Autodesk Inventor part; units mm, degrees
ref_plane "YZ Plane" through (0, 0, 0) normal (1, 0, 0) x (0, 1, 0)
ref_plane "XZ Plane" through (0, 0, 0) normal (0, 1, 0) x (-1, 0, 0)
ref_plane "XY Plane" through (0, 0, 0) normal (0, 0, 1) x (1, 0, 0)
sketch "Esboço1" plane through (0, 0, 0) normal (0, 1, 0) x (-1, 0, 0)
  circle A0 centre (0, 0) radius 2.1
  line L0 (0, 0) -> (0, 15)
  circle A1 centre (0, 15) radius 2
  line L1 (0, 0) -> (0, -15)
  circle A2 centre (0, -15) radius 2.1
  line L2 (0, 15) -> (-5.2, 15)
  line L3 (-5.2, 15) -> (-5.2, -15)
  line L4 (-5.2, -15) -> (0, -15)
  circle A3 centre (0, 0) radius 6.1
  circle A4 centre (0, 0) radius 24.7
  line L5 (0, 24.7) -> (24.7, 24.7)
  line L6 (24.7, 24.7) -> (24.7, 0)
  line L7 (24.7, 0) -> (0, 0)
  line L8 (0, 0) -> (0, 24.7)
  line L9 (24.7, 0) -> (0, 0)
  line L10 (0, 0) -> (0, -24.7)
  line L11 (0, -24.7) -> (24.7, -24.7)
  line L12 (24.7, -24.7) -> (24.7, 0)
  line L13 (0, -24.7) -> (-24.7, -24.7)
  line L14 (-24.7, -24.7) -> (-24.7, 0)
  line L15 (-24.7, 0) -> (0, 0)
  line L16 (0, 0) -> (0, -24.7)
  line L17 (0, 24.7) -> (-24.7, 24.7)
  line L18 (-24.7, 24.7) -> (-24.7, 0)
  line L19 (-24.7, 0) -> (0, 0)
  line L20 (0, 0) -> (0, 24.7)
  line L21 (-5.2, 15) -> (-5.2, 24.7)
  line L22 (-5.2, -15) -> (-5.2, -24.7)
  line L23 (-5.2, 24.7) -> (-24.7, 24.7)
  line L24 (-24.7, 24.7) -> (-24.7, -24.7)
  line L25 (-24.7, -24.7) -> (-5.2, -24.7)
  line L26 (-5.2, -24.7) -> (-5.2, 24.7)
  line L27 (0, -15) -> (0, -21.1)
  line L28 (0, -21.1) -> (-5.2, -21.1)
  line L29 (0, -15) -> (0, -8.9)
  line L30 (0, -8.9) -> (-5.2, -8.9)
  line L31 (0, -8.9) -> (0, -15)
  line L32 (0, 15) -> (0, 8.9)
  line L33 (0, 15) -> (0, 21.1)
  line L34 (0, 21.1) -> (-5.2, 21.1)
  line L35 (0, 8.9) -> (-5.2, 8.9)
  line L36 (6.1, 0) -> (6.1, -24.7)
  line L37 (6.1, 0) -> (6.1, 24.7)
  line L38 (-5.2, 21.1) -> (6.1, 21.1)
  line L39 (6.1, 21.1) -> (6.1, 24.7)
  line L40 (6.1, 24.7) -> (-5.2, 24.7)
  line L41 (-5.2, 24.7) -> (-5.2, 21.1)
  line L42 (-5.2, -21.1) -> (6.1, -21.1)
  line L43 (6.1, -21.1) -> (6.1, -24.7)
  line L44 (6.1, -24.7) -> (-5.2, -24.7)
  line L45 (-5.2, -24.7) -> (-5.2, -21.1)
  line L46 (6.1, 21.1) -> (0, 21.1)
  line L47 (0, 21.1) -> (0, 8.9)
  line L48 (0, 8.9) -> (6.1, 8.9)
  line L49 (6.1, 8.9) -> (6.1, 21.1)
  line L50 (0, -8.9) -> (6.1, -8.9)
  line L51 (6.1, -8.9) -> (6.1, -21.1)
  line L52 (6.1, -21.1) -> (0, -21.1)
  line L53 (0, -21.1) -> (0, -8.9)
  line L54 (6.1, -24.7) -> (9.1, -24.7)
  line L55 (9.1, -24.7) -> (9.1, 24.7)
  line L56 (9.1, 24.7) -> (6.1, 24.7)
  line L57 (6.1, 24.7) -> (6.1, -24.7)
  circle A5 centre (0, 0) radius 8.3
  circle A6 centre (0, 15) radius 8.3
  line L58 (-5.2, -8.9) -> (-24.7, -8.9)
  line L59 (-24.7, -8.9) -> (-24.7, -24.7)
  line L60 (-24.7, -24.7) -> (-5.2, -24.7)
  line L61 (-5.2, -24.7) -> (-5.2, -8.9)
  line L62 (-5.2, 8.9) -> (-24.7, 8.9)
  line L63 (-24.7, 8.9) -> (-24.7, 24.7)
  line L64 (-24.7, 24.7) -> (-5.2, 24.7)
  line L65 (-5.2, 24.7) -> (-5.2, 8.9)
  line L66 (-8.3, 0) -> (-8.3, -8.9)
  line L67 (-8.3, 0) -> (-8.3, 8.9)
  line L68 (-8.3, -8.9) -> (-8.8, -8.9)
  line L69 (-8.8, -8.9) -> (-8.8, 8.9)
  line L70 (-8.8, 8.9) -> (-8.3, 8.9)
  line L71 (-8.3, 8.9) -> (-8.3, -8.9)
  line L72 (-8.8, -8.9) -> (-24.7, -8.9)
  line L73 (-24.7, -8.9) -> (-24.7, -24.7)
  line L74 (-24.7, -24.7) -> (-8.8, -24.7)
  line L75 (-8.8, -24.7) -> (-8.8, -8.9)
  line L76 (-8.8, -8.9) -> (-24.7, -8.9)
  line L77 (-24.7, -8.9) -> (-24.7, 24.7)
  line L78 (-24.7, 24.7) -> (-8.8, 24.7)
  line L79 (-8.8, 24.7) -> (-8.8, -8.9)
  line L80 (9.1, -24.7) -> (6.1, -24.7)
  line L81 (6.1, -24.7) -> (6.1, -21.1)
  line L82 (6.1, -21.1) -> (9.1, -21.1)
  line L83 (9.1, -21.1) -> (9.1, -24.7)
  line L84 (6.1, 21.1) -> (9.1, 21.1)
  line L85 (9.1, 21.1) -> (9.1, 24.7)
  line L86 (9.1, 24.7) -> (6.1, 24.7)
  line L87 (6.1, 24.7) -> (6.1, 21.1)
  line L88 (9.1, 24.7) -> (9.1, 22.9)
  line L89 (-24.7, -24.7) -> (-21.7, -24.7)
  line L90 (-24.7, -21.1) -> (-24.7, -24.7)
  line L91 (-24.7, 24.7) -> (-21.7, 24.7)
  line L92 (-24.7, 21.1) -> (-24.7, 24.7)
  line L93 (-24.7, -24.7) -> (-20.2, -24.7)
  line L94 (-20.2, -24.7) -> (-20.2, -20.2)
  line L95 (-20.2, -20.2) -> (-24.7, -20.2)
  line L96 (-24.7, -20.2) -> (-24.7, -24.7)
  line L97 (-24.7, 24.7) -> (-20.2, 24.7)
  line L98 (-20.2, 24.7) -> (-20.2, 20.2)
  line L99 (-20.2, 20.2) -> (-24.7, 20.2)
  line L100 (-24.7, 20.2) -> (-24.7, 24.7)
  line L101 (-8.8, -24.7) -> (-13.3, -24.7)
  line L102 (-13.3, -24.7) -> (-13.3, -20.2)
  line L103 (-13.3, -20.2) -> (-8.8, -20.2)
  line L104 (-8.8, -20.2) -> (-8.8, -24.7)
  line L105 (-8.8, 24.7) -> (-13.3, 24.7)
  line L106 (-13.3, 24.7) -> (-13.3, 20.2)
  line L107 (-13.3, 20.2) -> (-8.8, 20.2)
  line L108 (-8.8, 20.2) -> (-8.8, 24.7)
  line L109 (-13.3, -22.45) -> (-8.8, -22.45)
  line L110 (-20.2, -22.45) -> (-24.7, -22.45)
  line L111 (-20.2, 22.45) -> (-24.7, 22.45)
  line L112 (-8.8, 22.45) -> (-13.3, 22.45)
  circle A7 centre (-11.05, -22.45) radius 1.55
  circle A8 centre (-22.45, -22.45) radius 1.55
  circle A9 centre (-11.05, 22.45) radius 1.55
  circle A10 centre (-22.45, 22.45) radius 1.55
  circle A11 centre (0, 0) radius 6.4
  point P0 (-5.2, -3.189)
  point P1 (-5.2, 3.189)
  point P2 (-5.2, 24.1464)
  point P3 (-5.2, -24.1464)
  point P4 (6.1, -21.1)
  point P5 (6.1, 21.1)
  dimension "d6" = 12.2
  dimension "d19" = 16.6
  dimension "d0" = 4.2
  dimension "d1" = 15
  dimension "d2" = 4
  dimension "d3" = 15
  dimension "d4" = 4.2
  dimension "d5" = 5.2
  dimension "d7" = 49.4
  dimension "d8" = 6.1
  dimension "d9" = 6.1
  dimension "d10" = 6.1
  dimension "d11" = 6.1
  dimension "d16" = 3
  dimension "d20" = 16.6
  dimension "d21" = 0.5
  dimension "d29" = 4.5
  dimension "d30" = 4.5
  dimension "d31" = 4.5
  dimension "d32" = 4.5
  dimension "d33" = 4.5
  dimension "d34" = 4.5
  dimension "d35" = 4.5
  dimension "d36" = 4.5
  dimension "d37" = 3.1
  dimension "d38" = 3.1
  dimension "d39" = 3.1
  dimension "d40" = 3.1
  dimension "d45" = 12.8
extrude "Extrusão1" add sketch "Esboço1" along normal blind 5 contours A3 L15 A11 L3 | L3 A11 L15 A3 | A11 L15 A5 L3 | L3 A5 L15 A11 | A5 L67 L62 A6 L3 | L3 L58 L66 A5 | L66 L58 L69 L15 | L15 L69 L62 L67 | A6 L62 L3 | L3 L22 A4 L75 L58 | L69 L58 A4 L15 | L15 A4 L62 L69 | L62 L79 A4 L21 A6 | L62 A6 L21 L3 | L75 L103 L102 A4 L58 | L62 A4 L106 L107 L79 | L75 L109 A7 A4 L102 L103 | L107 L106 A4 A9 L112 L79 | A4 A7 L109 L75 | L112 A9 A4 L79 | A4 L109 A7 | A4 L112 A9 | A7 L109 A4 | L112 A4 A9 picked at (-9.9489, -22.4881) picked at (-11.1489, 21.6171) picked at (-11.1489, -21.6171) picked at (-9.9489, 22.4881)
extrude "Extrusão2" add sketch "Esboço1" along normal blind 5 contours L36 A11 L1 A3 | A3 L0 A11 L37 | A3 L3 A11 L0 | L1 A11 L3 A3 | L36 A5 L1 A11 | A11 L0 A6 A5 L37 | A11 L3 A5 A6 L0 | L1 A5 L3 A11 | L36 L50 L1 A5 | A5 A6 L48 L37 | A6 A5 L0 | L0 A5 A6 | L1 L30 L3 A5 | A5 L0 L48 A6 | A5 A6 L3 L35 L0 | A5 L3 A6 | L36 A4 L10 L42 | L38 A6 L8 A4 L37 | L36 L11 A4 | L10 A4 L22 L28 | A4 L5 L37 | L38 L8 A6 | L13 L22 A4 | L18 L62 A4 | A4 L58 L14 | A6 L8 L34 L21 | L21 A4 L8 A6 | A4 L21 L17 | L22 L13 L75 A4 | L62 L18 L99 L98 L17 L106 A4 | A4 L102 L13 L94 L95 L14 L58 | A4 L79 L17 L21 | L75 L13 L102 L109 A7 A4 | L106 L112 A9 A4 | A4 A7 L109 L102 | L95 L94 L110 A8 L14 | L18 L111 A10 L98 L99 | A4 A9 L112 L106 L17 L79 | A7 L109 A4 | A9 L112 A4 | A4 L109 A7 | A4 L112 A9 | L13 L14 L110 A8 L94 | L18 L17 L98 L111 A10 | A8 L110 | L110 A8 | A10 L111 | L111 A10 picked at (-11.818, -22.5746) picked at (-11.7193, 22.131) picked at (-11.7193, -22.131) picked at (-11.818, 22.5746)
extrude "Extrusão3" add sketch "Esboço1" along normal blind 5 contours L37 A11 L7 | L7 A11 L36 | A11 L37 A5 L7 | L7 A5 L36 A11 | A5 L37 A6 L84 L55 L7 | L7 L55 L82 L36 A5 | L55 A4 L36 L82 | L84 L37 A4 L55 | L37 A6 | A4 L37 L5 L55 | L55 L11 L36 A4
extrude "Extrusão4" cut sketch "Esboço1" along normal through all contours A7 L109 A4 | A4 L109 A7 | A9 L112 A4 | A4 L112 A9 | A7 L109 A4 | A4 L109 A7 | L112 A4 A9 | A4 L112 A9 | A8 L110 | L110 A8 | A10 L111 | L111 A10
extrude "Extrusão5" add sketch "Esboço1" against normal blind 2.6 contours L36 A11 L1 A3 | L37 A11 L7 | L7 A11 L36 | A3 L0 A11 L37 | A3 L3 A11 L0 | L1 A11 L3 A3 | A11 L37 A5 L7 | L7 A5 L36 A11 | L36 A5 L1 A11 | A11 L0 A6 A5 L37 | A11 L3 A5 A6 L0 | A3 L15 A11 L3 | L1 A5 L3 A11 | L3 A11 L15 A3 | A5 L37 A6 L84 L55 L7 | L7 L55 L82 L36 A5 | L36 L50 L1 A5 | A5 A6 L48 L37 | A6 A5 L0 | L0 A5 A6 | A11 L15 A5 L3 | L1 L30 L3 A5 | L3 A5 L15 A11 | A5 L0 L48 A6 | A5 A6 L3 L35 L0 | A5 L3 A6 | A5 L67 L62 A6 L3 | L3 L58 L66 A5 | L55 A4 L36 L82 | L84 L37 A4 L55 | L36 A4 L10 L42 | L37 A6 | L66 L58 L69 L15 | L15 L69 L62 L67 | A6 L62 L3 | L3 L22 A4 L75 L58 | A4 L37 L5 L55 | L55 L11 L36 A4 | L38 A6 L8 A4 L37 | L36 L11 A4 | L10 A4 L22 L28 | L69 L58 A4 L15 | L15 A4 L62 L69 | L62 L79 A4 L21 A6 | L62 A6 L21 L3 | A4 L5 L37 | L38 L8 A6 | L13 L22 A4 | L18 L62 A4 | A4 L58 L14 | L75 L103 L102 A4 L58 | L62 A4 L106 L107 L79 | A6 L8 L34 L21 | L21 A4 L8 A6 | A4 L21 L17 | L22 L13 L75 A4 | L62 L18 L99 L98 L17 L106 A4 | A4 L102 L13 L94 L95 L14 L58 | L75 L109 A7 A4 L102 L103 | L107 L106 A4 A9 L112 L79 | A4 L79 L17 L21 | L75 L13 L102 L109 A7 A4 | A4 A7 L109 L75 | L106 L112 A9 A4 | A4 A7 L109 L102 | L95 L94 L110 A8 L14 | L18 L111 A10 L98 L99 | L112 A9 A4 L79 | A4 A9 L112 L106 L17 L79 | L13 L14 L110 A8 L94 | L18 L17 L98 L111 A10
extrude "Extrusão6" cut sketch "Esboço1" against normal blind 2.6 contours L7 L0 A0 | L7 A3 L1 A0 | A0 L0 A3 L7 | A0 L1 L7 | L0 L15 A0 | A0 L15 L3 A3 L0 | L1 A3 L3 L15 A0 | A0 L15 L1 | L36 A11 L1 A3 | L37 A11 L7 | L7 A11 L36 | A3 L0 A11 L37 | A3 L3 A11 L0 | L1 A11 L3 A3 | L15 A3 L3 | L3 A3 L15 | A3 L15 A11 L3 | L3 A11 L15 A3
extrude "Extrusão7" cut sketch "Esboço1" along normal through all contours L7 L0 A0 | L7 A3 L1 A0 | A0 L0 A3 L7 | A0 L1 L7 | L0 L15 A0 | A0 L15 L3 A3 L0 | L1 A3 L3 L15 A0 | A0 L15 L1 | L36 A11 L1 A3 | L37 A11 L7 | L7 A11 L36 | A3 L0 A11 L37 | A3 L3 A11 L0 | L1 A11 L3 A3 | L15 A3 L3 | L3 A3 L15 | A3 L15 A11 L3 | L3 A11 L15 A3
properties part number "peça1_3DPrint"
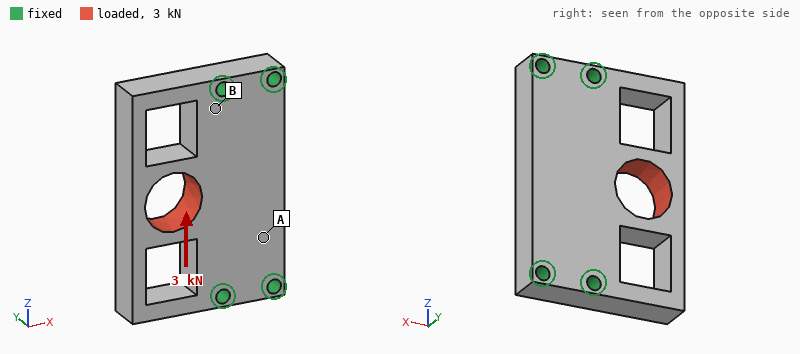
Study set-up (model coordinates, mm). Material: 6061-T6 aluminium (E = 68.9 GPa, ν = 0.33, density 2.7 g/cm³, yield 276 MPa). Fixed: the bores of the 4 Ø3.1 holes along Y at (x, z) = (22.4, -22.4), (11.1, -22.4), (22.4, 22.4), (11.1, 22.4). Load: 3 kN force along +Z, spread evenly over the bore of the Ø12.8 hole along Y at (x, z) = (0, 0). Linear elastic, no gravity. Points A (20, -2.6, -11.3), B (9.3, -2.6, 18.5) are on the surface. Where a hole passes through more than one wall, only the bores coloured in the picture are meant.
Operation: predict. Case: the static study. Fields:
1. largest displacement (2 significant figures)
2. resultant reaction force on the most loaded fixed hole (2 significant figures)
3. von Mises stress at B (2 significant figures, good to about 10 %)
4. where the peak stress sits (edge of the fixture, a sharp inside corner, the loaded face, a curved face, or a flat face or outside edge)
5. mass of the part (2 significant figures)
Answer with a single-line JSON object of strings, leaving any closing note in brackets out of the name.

{"largest displacement": "59 µm", "resultant reaction force on the most loaded fixed hole": "1.2 kN", "von Mises stress at B": "31 MPa", "where the peak stress sits": "the loaded face", "mass of the part": "25 g"}
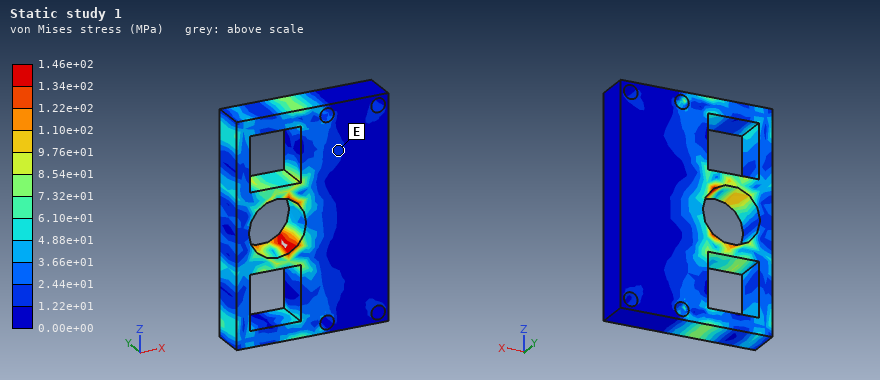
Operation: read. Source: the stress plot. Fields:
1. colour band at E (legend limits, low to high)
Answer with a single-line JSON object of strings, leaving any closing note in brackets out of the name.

{"colour band at E": "1.22e+01 to 2.44e+01 MPa"}
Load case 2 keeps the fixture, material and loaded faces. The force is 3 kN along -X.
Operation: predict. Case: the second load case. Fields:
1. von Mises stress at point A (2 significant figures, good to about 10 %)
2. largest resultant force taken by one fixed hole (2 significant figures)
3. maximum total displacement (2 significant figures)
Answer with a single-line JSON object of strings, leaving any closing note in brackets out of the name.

{"von Mises stress at point A": "18 MPa", "largest resultant force taken by one fixed hole": "1.3 kN", "maximum total displacement": "26 µm"}
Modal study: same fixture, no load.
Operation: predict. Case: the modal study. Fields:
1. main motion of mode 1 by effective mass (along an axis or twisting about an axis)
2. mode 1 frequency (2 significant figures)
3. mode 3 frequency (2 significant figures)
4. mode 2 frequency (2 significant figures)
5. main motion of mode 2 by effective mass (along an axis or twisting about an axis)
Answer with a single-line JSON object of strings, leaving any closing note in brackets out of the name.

{"main motion of mode 1 by effective mass": "along Y", "mode 1 frequency": "8900 Hz", "mode 3 frequency": "14 kHz", "mode 2 frequency": "13 kHz", "main motion of mode 2 by effective mass": "along Z"}
